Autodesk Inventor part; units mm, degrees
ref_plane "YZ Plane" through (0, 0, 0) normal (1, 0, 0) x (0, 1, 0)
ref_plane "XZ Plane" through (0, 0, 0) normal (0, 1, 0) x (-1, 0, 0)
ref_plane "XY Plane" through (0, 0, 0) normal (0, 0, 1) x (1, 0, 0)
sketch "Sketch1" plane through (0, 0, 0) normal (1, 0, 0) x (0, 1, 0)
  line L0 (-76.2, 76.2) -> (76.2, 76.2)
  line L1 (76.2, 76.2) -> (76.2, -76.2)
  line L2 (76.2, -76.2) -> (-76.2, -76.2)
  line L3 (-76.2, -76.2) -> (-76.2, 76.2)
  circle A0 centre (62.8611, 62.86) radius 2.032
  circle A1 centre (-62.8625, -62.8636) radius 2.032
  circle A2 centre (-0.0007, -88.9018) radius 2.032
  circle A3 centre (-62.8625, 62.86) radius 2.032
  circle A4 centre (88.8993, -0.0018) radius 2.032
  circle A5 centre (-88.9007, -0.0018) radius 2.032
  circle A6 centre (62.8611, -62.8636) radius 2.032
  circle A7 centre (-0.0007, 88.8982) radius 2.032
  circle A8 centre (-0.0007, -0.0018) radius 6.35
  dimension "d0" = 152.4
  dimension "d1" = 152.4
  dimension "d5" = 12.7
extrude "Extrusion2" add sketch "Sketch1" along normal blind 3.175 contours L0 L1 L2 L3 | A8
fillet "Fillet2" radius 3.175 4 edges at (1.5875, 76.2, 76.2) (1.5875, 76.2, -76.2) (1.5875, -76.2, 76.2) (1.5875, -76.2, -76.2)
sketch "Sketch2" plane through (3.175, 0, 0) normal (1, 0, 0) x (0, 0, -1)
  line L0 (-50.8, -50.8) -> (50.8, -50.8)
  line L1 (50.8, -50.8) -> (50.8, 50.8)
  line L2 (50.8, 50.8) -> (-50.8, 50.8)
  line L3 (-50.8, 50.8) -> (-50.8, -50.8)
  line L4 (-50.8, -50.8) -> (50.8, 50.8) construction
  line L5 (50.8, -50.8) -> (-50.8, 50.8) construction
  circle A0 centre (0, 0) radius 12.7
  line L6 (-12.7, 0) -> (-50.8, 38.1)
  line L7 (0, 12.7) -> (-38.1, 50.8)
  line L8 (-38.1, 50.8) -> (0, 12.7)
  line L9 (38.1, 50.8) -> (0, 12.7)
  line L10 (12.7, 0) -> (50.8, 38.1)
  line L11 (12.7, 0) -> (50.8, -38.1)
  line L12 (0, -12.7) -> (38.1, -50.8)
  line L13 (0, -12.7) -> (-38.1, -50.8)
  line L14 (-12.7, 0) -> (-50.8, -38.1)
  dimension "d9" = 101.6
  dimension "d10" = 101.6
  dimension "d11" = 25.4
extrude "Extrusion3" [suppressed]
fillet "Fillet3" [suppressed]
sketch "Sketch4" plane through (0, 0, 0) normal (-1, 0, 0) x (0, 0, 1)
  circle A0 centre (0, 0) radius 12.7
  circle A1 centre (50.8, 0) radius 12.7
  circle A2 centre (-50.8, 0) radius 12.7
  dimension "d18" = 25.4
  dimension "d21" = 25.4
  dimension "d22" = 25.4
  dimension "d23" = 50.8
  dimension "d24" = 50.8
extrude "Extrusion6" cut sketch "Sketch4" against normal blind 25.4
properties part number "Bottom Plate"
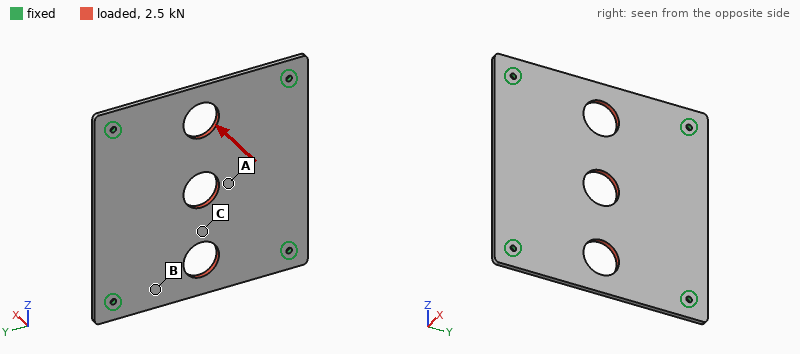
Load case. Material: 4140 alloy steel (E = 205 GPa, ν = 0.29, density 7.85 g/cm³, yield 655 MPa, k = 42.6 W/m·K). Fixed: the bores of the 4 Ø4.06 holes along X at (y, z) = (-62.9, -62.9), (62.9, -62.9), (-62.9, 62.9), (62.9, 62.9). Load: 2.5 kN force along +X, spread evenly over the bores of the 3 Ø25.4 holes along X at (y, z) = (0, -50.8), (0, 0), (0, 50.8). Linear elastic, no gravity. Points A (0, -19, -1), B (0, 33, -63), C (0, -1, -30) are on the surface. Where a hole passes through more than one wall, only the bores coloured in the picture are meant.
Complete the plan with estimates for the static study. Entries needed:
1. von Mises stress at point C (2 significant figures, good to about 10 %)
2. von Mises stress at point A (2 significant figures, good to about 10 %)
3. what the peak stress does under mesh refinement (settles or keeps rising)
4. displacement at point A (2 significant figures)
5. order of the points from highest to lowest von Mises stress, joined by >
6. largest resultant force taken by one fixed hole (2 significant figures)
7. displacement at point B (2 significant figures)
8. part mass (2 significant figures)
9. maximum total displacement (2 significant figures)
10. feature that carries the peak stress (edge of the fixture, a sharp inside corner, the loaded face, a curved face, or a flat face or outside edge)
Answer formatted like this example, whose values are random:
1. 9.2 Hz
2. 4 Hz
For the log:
1. 250 MPa
2. 100 MPa
3. keeps rising
4. 0.73 mm
5. C > A > B
6. 630 N
7. 0.28 mm
8. 540 g
9. 0.84 mm
10. edge of the fixture
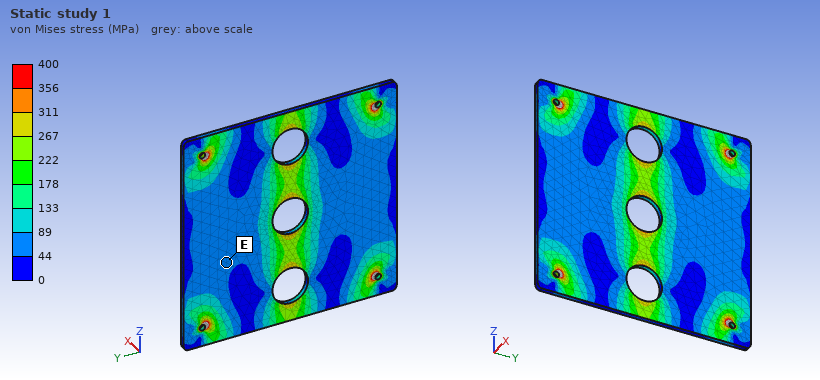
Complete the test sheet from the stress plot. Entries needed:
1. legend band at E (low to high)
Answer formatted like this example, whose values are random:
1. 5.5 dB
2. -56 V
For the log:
1. 44 to 89 MPa
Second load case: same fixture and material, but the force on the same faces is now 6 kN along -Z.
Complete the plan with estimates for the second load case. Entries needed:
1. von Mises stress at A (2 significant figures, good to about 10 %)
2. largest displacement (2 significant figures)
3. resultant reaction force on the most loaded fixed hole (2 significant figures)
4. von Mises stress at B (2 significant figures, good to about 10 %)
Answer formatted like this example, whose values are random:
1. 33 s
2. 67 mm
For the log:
1. 15 MPa
2. 8.6 µm
3. 1.6 kN
4. 7.1 MPa
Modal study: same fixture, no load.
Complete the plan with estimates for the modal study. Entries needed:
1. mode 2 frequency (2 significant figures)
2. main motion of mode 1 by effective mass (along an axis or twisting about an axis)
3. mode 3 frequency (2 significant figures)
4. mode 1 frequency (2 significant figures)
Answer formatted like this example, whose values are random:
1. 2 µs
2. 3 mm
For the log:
1. 1100 Hz
2. along X
3. 1100 Hz
4. 660 Hz
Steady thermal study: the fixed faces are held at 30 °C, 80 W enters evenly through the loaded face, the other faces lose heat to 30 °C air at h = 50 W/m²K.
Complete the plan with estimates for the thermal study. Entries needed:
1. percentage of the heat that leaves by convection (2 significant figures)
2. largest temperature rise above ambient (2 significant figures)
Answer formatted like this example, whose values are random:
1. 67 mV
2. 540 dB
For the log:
1. 81 %
2. 72 K
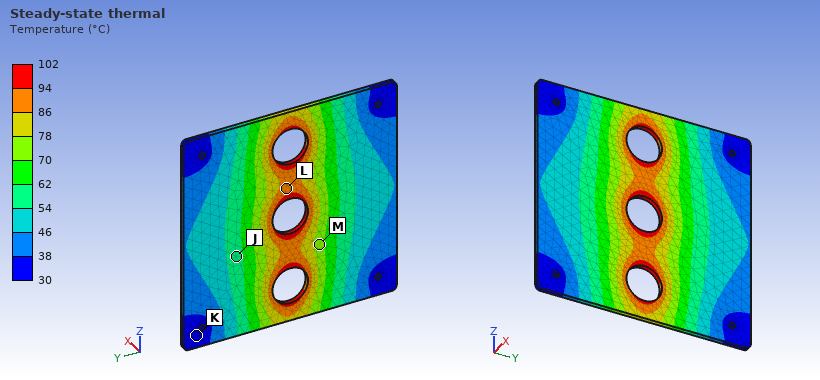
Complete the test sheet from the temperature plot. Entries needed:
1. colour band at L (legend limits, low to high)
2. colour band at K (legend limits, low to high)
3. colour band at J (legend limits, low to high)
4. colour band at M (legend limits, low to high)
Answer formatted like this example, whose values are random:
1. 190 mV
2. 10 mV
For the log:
1. 86 to 94 °C
2. 30 to 38 °C
3. 54 to 62 °C
4. 70 to 78 °C
